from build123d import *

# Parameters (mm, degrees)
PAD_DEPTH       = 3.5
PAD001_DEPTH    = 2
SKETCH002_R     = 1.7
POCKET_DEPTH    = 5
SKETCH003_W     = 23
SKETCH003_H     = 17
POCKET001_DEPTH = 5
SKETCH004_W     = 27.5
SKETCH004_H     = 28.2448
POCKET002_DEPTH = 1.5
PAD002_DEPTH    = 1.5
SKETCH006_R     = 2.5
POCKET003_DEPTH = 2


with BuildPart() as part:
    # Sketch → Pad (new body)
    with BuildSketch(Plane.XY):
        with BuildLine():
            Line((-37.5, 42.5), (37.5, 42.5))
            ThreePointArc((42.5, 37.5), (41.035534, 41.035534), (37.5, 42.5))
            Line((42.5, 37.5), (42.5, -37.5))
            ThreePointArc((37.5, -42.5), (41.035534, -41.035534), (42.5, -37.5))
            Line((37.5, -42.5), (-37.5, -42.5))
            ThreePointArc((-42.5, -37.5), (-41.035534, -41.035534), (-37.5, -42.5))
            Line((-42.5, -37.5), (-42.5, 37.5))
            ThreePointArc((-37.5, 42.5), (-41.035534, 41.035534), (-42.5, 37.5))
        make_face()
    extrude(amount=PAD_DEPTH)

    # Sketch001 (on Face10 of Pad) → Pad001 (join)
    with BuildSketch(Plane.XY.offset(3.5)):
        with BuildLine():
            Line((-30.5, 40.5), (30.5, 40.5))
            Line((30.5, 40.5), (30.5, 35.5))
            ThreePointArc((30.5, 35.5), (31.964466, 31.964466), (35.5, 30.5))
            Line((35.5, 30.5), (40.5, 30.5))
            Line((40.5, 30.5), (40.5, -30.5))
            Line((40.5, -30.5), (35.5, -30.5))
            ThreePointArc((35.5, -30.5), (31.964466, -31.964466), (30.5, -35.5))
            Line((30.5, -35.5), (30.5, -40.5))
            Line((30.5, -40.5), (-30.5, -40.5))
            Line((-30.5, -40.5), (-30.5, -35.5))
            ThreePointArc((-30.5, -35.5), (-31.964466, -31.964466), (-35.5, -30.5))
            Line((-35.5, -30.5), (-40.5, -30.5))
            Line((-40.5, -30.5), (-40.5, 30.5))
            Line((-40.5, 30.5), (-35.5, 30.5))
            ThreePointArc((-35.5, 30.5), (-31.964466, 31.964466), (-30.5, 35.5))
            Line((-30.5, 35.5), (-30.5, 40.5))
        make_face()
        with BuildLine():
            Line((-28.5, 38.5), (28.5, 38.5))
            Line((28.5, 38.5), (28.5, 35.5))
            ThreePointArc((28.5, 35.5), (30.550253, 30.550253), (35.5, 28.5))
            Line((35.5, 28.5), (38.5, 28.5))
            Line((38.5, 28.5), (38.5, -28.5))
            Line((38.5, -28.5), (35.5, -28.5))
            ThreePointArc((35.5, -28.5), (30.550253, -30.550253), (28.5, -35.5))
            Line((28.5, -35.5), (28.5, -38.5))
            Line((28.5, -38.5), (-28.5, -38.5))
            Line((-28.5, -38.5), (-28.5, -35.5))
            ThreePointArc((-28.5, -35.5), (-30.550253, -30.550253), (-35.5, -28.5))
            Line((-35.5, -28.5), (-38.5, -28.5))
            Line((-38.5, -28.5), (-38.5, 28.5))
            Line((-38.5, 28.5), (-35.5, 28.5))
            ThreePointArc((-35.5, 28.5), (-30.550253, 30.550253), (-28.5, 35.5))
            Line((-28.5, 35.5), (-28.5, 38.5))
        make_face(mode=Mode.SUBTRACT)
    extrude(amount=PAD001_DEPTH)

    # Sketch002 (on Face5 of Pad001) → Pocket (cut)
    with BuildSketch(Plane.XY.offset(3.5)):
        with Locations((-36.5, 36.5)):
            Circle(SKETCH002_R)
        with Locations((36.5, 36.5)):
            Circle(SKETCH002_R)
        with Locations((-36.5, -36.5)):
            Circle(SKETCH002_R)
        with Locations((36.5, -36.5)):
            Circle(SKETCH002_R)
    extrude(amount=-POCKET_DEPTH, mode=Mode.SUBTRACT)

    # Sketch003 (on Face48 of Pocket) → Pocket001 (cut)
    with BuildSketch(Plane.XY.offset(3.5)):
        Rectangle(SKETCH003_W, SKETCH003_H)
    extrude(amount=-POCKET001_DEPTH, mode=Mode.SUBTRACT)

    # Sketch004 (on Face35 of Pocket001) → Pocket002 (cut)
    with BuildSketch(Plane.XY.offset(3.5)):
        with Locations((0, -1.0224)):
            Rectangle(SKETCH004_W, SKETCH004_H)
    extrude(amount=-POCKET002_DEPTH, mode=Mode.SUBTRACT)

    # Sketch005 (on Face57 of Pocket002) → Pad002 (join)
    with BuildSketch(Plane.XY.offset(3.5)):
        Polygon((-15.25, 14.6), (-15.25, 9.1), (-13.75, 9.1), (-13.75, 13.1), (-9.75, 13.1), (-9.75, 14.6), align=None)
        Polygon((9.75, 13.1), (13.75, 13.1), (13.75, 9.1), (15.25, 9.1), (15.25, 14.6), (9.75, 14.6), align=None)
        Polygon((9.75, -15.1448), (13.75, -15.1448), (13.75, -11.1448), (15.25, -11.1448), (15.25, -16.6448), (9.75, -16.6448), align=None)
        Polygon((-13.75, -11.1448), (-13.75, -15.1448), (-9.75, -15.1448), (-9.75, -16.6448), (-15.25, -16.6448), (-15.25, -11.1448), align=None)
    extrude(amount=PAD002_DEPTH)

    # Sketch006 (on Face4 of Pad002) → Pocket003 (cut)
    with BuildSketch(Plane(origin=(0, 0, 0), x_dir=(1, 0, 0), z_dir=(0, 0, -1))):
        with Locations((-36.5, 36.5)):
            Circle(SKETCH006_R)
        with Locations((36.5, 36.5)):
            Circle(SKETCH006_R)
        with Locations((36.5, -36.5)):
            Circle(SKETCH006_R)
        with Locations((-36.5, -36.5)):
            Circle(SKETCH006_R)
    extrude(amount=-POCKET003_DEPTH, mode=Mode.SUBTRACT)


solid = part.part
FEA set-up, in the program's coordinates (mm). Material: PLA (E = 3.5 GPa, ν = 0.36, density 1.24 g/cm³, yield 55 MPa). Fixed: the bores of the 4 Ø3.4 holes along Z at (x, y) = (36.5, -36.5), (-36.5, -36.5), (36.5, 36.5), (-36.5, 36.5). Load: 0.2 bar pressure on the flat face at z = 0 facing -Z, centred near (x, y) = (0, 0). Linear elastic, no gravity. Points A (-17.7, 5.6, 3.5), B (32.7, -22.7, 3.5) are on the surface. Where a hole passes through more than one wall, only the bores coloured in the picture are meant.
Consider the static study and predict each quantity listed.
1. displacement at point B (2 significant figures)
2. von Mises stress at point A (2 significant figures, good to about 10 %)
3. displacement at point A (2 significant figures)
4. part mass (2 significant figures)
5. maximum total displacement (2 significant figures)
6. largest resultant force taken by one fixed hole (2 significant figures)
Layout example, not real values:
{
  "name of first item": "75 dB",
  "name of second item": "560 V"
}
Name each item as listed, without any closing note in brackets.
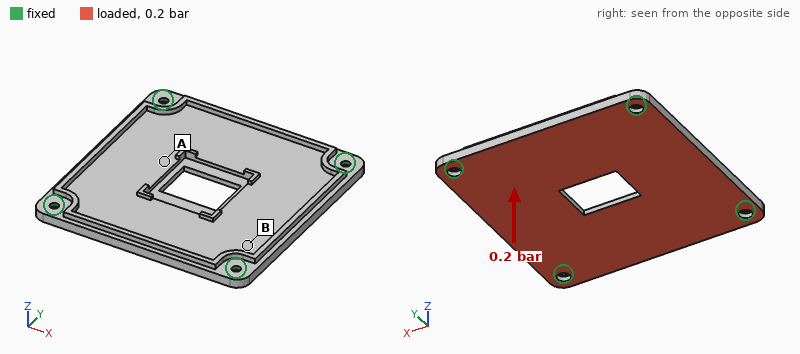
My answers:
{
  "displacement at point B": "0.14 mm",
  "von Mises stress at point A": "3.3 MPa",
  "displacement at point A": "0.40 mm",
  "part mass": "30 g",
  "maximum total displacement": "0.51 mm",
  "largest resultant force taken by one fixed hole": "69 N"
}
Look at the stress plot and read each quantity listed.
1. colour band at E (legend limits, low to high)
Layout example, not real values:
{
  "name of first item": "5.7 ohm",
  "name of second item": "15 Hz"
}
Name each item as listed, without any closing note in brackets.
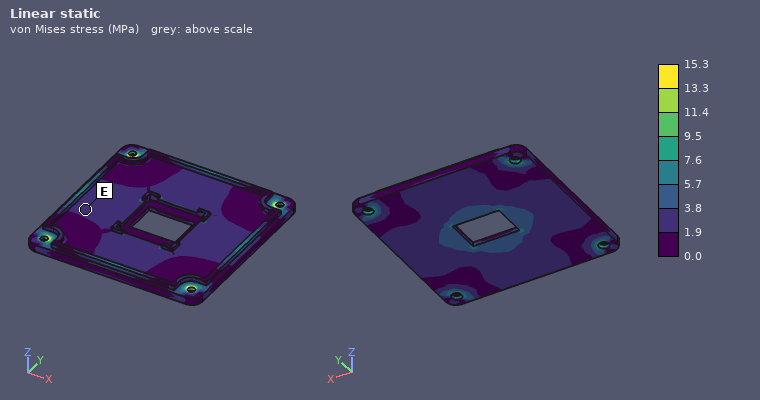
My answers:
{
  "colour band at E": "1.9 to 3.8 MPa"
}
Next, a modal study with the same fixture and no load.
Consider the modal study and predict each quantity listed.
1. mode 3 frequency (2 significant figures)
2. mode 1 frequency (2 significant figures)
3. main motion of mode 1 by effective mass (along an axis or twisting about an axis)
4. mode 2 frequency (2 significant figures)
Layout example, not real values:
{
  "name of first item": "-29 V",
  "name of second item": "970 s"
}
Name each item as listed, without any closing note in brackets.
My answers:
{
  "mode 3 frequency": "1100 Hz",
  "mode 1 frequency": "640 Hz",
  "main motion of mode 1 by effective mass": "along Z",
  "mode 2 frequency": "1100 Hz"
}
